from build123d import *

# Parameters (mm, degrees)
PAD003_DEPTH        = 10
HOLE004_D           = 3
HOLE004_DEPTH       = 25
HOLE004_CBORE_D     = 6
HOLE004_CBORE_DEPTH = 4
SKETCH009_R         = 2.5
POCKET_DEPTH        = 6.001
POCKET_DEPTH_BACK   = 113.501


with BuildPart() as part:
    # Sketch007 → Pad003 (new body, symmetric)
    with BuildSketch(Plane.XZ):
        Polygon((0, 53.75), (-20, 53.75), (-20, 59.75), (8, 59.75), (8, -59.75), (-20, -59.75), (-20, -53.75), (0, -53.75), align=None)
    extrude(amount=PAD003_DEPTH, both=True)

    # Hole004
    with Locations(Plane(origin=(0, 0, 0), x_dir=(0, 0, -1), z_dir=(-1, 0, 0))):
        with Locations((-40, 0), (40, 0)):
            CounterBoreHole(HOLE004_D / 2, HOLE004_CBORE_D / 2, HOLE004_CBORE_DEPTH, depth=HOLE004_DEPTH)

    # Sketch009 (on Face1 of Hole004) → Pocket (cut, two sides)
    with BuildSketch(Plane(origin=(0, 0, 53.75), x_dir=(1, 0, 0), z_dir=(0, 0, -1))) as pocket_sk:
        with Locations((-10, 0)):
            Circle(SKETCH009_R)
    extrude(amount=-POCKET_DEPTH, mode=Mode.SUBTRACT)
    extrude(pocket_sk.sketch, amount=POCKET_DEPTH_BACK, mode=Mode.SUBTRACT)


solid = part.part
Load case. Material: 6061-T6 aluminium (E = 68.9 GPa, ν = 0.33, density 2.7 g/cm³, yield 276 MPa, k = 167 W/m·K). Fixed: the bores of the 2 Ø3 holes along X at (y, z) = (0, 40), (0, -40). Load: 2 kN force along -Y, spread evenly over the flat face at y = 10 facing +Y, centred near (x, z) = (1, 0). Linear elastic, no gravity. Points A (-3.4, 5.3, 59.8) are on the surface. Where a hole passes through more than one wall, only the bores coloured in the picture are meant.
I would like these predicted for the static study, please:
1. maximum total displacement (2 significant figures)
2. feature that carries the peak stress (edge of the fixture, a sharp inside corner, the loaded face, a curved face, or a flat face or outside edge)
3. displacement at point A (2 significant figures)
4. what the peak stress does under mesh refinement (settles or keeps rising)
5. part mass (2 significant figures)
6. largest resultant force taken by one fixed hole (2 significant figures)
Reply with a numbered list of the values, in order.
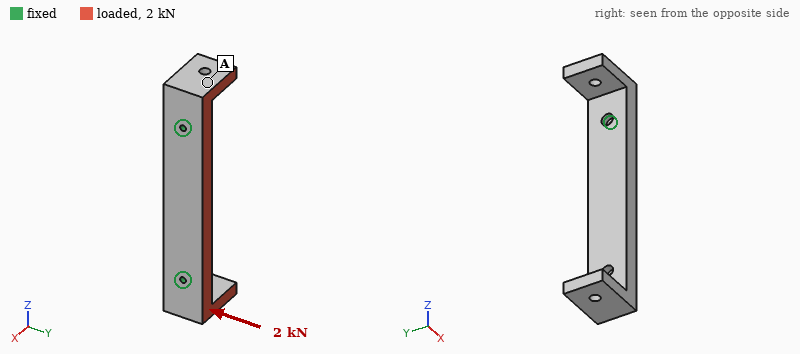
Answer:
1. 64 µm
2. edge of the fixture
3. 25 µm
4. keeps rising
5. 63 g
6. 1.0 kN
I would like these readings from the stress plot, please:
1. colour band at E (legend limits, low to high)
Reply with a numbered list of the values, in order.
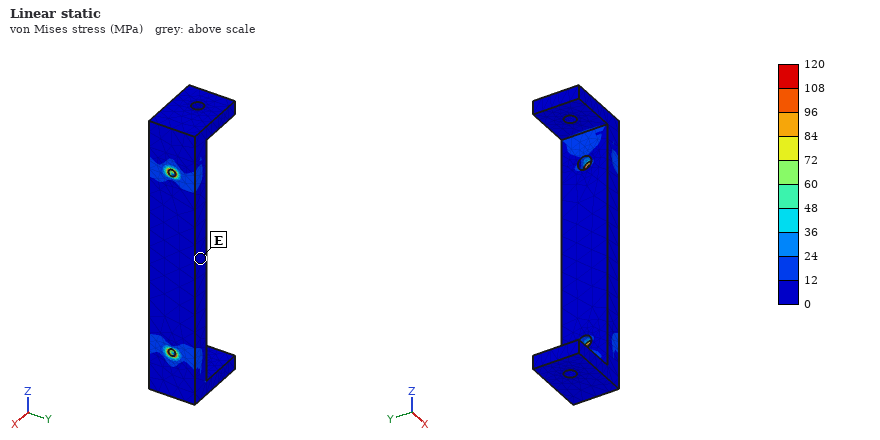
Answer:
1. 0 to 12 MPa
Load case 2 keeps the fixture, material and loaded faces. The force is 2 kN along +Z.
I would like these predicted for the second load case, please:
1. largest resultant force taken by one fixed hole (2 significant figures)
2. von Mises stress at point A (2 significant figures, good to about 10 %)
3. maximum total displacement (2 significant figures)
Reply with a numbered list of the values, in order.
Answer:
1. 1.0 kN
2. 17 MPa
3. 69 µm
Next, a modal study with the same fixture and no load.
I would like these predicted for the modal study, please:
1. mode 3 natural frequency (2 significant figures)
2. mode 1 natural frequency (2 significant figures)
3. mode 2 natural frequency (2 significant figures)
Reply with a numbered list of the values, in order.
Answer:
1. 4100 Hz
2. 3400 Hz
3. 4100 Hz
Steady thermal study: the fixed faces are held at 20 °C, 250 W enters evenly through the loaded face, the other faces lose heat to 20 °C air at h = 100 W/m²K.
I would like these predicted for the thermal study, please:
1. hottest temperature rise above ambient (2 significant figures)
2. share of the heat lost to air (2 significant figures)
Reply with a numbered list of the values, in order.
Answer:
1. 75 K
2. 16 %
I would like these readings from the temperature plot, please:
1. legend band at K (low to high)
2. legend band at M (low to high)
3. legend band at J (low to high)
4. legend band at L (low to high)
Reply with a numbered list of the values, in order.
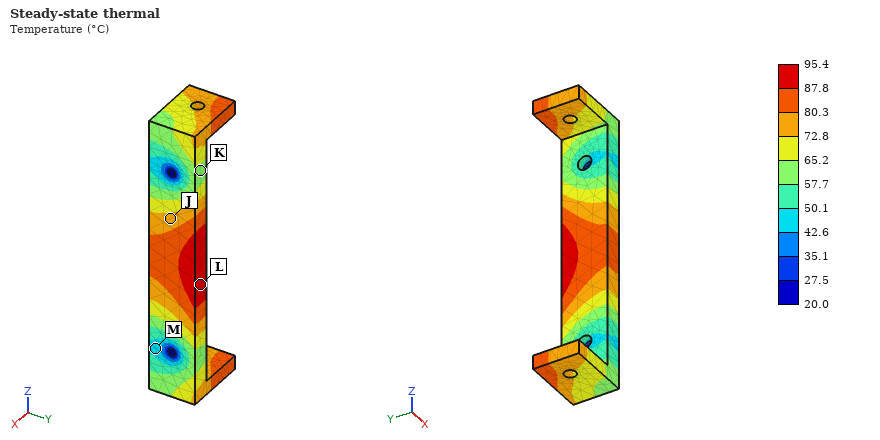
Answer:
1. 57.7 to 65.2 °C
2. 42.6 to 50.1 °C
3. 72.8 to 80.3 °C
4. 87.8 to 95.4 °C
